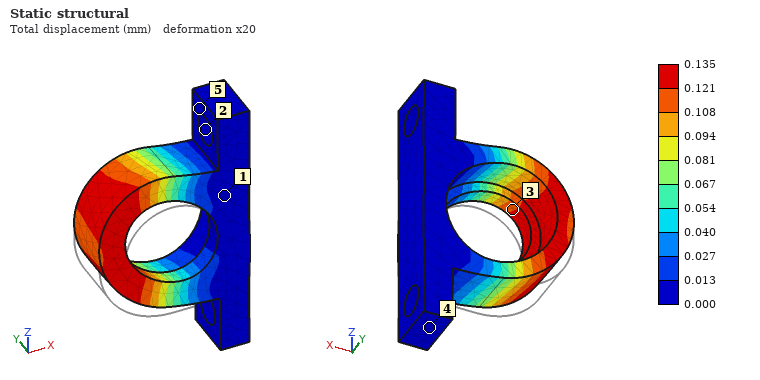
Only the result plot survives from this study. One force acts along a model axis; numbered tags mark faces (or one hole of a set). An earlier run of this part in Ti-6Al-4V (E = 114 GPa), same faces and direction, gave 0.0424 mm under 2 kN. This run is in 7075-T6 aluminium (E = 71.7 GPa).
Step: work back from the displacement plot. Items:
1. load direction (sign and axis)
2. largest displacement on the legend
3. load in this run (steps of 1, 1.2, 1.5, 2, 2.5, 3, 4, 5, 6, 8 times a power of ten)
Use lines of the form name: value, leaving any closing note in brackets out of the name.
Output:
load direction: +Z
largest displacement on the legend: 0.135 mm
load in this run: 4 kN
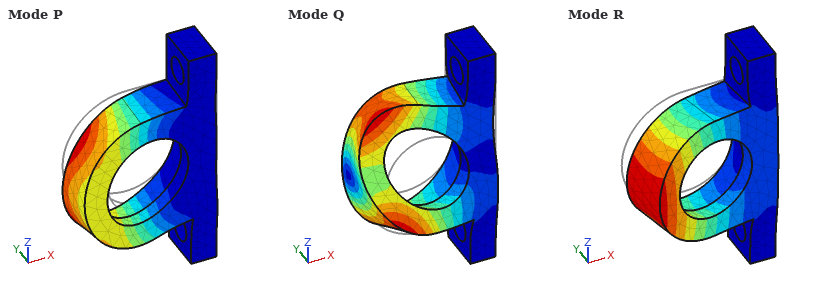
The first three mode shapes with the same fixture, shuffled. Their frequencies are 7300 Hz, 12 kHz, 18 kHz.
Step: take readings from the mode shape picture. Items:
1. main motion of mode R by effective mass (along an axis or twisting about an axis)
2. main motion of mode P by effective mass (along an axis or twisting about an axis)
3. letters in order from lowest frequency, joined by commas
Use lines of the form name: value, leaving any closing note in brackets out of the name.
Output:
main motion of mode R by effective mass: along Y
main motion of mode P by effective mass: along Z
letters in order from lowest frequency, joined by commas: R, P, Q
